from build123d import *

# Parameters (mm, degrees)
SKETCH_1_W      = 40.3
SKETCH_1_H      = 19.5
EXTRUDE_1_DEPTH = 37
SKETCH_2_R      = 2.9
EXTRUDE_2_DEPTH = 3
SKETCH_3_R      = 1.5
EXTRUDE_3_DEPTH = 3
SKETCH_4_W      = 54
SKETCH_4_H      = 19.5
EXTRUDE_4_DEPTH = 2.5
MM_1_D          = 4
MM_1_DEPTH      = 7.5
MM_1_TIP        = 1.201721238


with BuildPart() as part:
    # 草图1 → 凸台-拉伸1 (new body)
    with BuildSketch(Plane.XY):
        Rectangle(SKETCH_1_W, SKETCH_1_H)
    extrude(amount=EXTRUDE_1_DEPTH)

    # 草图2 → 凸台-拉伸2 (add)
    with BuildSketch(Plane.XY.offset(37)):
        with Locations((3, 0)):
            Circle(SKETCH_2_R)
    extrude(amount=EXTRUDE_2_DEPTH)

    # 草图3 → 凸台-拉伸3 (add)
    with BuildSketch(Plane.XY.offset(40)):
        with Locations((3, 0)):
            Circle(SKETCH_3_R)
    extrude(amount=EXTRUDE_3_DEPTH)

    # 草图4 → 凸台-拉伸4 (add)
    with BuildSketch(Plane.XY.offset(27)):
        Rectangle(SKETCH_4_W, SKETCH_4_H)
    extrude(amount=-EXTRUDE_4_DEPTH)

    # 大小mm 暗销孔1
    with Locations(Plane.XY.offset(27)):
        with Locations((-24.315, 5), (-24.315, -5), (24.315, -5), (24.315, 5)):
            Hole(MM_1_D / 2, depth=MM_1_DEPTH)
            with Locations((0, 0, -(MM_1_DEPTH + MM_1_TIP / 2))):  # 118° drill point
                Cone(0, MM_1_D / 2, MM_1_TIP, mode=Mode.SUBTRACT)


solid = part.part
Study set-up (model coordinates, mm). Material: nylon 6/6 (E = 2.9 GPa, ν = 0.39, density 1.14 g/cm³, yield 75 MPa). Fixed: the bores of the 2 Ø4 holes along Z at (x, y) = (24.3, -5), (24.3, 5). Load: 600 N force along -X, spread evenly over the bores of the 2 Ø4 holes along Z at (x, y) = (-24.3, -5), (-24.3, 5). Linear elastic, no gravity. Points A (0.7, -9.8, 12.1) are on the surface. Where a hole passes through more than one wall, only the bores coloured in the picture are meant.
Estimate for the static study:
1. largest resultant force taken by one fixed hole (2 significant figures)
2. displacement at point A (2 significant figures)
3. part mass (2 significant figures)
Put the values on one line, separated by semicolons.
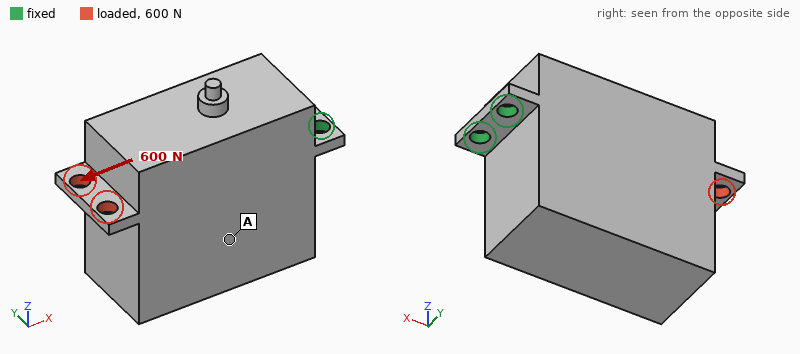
300 N; 0.034 mm; 34 g
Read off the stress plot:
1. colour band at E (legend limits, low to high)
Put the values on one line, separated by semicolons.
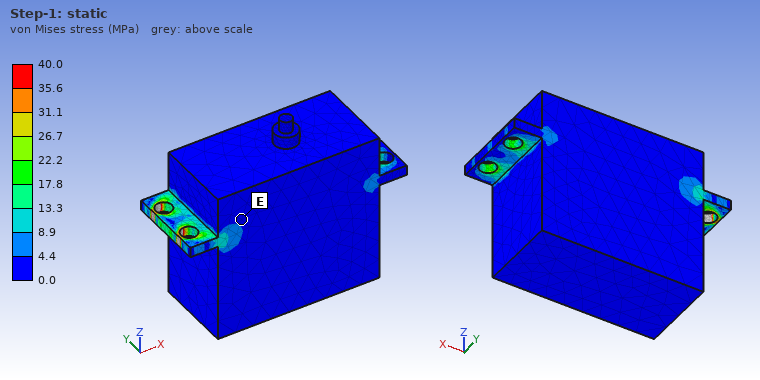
0.0 to 4.4 MPa
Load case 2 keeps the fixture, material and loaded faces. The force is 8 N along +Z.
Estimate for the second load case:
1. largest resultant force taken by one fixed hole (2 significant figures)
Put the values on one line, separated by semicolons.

4.0 N
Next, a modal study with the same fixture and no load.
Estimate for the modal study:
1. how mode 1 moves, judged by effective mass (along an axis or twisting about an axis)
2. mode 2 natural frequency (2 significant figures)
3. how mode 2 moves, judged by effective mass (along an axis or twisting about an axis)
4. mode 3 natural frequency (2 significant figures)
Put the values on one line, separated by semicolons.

along Z; 700 Hz; along Y; 1100 Hz
